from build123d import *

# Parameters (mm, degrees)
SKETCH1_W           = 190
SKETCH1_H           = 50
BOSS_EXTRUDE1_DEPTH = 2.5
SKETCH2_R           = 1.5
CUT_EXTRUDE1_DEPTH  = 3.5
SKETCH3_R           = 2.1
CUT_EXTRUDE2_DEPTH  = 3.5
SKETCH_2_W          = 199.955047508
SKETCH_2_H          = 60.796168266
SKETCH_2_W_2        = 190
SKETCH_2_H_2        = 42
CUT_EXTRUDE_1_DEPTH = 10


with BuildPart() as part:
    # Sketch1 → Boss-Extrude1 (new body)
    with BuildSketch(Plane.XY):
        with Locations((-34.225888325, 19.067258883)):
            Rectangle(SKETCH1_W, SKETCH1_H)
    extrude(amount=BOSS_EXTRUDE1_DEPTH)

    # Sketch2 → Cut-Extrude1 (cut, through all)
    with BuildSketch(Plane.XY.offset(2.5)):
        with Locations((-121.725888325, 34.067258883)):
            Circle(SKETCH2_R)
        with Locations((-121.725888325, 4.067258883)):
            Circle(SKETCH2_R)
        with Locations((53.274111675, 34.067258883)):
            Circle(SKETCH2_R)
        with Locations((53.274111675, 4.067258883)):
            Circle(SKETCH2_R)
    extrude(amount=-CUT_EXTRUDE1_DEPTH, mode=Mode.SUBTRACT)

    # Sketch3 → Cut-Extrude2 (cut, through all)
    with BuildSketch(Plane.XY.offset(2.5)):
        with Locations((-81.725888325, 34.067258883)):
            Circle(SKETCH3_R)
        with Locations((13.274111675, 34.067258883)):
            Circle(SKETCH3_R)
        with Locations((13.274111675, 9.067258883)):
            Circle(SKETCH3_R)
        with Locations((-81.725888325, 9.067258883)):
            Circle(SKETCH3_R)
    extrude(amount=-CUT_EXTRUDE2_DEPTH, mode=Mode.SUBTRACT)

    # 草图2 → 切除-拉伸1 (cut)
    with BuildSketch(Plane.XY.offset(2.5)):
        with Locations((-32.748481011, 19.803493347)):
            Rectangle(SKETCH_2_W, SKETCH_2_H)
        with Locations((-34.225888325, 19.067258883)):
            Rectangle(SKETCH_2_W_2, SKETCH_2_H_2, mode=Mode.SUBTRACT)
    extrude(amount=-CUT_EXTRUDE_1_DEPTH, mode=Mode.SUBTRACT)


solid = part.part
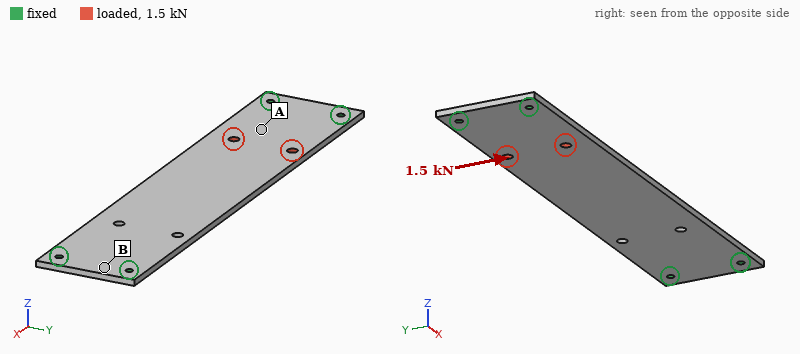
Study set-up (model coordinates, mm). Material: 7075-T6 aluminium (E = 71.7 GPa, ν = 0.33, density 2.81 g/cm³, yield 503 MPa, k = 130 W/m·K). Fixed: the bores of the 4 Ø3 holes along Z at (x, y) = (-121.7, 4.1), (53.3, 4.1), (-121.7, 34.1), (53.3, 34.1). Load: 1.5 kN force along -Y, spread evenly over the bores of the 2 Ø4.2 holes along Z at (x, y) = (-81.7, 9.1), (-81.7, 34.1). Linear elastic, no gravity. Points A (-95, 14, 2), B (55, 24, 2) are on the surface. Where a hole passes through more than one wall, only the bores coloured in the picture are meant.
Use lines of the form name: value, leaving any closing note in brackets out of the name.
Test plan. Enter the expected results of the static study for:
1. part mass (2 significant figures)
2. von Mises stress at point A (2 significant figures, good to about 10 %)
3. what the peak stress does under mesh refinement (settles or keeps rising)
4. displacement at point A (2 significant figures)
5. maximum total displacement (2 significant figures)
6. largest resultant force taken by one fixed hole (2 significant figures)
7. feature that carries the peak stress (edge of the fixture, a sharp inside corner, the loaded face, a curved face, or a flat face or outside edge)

part mass: 55 g
von Mises stress at point A: 29 MPa
what the peak stress does under mesh refinement: keeps rising
displacement at point A: 24 µm
maximum total displacement: 39 µm
largest resultant force taken by one fixed hole: 1.2 kN
feature that carries the peak stress: edge of the fixture
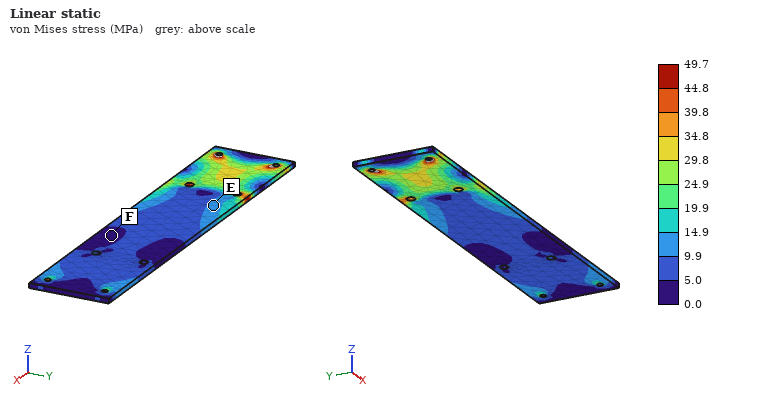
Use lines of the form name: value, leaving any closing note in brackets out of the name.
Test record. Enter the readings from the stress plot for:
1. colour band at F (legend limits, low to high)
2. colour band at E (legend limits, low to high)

colour band at F: 0.0 to 5.0 MPa
colour band at E: 9.9 to 14.9 MPa
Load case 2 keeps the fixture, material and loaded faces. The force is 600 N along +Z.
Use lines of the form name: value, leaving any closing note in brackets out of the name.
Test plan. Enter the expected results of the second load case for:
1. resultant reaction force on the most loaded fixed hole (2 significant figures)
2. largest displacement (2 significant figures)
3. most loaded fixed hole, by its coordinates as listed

resultant reaction force on the most loaded fixed hole: 300 N
largest displacement: 2.3 mm
most loaded fixed hole, by its coordinates as listed: (-121.7, 34.1)
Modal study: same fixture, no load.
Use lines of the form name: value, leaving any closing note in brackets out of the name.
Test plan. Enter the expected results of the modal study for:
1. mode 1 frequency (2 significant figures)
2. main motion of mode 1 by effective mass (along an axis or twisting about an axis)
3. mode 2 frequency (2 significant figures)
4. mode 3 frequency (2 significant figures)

mode 1 frequency: 420 Hz
main motion of mode 1 by effective mass: along Z
mode 2 frequency: 1200 Hz
mode 3 frequency: 1200 Hz
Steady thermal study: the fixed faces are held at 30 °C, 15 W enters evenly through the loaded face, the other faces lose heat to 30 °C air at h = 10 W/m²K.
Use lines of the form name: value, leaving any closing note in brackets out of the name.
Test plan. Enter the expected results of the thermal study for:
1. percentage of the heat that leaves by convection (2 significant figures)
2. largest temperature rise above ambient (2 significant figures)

percentage of the heat that leaves by convection: 16 %
largest temperature rise above ambient: 37 K
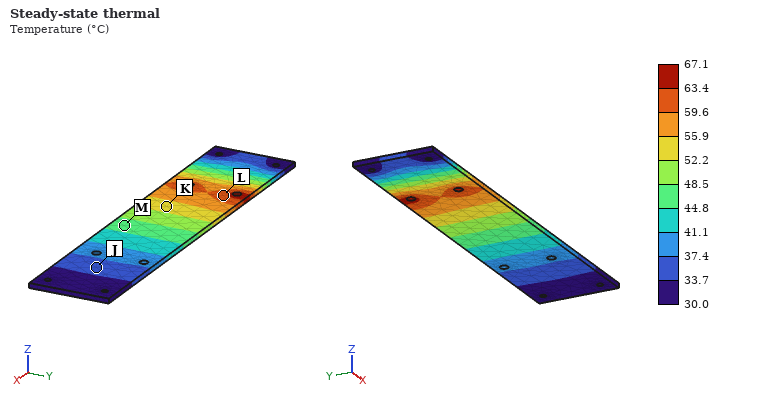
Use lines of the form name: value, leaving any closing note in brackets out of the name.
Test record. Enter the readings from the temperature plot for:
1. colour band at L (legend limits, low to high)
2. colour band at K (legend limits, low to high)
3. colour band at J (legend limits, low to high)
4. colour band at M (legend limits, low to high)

colour band at L: 59.6 to 63.4 °C
colour band at K: 52.2 to 55.9 °C
colour band at J: 33.7 to 37.4 °C
colour band at M: 44.8 to 48.5 °C
